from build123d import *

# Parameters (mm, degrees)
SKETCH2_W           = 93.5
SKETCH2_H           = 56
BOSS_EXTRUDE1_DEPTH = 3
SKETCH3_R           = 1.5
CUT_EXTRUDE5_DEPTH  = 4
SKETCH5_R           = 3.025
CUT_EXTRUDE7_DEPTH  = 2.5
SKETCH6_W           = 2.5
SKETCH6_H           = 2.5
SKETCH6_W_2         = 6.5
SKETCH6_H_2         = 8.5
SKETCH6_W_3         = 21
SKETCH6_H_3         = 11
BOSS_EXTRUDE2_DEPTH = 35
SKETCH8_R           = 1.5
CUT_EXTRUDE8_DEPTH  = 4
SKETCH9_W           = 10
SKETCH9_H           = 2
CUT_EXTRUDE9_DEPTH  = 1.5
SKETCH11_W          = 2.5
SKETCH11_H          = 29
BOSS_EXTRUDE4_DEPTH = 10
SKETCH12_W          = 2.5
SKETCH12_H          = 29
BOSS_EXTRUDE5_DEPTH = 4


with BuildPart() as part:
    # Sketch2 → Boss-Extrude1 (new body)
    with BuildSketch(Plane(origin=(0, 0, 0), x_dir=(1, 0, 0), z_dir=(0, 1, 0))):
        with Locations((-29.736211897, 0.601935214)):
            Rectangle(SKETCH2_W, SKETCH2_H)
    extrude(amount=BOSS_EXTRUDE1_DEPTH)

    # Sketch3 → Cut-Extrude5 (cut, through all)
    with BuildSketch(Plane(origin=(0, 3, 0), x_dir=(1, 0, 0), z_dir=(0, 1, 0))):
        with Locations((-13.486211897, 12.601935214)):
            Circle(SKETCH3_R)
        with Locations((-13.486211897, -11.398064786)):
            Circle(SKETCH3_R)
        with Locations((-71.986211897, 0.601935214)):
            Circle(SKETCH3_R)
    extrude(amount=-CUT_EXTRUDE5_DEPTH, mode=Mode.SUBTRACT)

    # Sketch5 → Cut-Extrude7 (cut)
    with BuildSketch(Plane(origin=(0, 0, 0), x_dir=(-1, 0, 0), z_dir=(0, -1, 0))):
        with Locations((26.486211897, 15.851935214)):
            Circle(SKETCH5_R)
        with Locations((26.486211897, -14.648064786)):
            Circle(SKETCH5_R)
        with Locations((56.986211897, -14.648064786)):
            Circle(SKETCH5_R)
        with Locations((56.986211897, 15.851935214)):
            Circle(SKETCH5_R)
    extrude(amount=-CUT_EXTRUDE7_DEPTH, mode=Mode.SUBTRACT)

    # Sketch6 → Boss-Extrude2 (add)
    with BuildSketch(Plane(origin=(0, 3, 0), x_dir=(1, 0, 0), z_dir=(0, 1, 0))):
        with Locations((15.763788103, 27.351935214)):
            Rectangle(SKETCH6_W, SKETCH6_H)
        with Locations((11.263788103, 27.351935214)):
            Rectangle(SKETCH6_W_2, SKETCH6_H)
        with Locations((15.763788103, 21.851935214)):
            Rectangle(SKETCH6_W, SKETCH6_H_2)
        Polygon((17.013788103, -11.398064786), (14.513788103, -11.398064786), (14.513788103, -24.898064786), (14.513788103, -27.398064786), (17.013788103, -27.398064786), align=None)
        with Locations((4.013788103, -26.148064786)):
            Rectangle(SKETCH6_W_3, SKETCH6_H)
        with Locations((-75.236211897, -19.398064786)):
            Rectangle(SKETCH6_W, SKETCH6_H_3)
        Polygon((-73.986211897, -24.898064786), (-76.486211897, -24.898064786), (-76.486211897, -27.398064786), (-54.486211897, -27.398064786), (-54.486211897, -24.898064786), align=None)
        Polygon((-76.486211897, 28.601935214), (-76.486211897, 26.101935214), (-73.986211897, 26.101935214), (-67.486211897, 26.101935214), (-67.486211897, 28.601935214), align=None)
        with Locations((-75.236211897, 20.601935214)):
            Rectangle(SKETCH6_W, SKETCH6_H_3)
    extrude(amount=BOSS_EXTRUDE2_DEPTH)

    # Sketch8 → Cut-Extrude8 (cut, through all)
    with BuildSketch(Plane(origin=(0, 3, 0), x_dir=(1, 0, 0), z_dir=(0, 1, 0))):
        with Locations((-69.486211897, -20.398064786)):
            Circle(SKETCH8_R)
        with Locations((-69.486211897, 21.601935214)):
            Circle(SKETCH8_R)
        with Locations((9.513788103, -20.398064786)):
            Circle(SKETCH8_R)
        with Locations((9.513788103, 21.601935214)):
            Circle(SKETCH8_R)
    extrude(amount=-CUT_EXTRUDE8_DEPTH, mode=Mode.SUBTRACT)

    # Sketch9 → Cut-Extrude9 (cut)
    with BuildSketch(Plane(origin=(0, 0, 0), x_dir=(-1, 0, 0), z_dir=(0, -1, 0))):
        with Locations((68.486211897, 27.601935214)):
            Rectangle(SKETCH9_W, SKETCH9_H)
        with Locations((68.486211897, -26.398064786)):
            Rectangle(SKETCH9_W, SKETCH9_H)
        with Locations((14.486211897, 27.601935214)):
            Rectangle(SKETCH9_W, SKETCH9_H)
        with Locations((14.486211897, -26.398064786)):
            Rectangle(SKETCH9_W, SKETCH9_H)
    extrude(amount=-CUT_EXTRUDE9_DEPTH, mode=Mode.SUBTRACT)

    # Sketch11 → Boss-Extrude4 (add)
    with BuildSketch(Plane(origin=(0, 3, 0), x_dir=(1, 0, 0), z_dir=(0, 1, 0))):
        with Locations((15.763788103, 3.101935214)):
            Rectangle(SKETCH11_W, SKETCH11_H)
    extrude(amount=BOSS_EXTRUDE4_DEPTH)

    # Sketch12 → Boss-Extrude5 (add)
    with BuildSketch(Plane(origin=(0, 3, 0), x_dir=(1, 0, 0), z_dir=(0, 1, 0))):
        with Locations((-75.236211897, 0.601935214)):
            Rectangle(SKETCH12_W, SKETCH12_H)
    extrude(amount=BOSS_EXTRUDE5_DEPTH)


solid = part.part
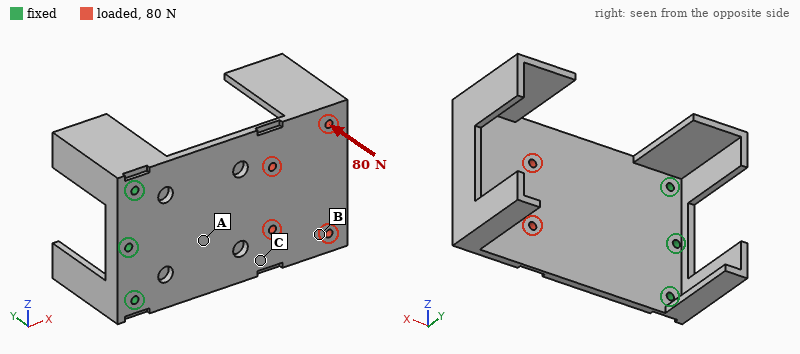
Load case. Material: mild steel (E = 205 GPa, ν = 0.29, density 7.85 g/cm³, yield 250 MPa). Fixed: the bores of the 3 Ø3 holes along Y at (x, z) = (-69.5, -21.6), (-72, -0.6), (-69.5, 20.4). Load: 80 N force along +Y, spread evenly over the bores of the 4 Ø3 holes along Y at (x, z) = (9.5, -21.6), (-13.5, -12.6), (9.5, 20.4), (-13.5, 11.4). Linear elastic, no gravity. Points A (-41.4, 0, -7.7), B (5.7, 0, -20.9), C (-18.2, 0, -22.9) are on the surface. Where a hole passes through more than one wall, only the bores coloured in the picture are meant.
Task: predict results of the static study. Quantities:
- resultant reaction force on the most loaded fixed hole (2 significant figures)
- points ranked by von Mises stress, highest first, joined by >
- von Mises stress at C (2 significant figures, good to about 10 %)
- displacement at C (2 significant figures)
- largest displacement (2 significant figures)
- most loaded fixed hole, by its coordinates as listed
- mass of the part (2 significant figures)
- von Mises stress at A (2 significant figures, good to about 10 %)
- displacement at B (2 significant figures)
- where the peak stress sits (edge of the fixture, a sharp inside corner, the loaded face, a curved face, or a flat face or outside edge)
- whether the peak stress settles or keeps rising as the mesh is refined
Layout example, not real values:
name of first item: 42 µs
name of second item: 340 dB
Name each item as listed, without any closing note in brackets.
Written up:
resultant reaction force on the most loaded fixed hole: 65 N
points ranked by von Mises stress, highest first, joined by >: A > C > B
von Mises stress at C: 19 MPa
displacement at C: 0.21 mm
largest displacement: 0.53 mm
most loaded fixed hole, by its coordinates as listed: (-72, -0.6)
mass of the part: 200 g
von Mises stress at A: 35 MPa
displacement at B: 0.37 mm
where the peak stress sits: edge of the fixture
whether the peak stress settles or keeps rising as the mesh is refined: keeps rising
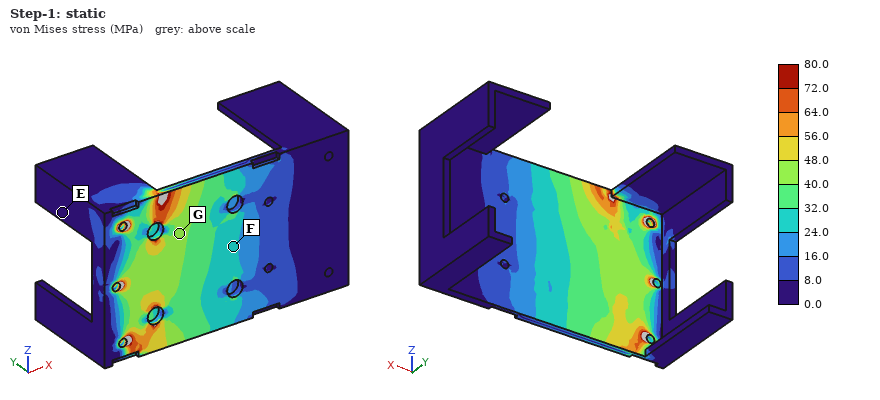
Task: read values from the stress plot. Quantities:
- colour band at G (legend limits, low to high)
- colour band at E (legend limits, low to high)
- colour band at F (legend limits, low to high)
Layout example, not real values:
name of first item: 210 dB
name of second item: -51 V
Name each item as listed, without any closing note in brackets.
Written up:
colour band at G: 40.0 to 48.0 MPa
colour band at E: 0.0 to 8.0 MPa
colour band at F: 24.0 to 32.0 MPa
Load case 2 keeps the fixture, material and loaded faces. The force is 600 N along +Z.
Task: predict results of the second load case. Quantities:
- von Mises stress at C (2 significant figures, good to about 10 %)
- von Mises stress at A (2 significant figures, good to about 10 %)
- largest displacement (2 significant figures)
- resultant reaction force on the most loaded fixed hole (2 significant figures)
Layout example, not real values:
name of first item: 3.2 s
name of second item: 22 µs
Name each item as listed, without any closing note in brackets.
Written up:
von Mises stress at C: 7.8 MPa
von Mises stress at A: 8.5 MPa
largest displacement: 18 µm
resultant reaction force on the most loaded fixed hole: 980 N
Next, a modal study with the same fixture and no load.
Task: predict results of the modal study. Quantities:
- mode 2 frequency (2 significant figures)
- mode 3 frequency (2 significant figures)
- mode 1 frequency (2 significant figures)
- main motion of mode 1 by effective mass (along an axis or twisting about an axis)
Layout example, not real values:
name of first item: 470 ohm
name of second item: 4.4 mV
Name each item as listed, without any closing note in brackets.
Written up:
mode 2 frequency: 570 Hz
mode 3 frequency: 1100 Hz
mode 1 frequency: 210 Hz
main motion of mode 1 by effective mass: along Y
